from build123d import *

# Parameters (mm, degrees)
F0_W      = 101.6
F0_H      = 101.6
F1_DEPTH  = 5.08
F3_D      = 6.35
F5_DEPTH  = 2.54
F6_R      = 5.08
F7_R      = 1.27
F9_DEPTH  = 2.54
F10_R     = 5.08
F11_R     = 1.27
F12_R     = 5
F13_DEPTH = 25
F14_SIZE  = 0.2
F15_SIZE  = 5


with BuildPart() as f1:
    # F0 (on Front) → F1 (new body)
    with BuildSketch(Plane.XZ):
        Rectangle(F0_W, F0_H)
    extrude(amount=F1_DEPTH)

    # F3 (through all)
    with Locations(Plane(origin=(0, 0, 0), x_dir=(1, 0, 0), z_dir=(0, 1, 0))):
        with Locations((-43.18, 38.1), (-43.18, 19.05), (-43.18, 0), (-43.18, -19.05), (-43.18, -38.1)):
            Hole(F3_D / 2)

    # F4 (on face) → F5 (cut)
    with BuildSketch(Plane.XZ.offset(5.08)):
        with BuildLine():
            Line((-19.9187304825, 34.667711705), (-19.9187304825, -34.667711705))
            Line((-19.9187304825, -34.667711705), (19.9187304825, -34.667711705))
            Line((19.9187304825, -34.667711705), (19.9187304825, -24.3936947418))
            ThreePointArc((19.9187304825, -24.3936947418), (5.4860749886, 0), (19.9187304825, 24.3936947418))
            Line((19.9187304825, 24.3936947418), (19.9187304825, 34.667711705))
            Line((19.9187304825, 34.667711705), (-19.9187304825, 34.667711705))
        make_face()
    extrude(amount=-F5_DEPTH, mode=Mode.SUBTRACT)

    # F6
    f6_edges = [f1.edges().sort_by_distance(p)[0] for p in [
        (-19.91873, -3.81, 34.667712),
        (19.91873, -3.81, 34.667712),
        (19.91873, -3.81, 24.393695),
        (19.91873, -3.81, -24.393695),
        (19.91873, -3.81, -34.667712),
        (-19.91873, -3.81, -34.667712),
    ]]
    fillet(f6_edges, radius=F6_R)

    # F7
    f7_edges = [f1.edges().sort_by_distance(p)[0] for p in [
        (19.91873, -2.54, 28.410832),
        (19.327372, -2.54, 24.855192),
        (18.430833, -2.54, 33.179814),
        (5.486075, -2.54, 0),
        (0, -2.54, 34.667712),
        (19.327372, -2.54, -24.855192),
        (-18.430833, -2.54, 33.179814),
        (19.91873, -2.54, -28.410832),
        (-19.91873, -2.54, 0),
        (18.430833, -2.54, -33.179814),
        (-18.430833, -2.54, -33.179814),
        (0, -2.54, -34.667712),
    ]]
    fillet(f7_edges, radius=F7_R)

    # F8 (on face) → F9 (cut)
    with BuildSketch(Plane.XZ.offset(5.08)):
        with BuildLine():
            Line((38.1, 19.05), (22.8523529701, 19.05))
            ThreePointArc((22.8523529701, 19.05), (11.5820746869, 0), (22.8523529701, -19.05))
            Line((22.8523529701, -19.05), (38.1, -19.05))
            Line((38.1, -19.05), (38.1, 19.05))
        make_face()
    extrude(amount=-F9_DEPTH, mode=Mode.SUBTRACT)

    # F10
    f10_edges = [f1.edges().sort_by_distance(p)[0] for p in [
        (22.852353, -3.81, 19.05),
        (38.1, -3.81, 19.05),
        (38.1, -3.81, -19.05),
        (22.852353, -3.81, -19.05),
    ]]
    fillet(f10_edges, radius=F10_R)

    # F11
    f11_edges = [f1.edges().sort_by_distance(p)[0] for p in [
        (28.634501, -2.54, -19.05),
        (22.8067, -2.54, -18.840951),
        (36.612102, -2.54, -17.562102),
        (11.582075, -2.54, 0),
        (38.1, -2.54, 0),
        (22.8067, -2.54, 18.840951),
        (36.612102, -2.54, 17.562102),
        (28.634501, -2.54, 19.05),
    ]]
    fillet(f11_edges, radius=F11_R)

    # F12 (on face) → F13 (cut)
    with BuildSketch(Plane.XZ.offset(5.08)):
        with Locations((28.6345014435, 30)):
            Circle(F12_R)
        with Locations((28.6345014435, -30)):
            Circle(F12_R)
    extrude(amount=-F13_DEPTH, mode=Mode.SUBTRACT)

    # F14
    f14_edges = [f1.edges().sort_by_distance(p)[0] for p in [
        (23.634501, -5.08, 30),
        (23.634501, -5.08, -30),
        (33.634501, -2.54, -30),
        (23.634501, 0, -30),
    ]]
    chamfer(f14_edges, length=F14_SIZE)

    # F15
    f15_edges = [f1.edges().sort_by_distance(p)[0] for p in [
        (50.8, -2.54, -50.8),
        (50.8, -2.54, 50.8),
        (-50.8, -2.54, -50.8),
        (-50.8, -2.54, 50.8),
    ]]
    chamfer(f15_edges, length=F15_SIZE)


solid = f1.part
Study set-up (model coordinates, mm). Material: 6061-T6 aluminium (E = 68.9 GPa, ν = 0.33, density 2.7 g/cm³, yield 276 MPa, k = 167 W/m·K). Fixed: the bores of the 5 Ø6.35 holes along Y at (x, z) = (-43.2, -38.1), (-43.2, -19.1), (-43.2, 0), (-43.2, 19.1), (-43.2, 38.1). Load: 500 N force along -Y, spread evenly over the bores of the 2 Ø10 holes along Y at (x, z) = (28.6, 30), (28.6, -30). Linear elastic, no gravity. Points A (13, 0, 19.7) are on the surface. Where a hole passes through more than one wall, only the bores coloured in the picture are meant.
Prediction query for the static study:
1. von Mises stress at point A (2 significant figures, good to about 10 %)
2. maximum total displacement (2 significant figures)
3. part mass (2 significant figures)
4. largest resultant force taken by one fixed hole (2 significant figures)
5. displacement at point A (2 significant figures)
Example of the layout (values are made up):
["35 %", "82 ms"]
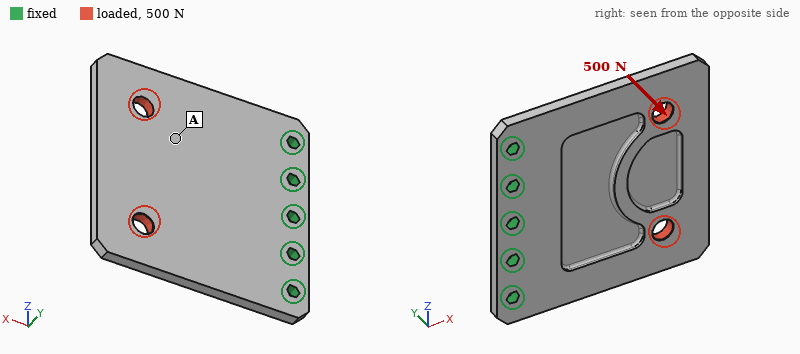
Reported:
["19 MPa", "1.6 mm", "120 g", "660 N", "0.70 mm"]
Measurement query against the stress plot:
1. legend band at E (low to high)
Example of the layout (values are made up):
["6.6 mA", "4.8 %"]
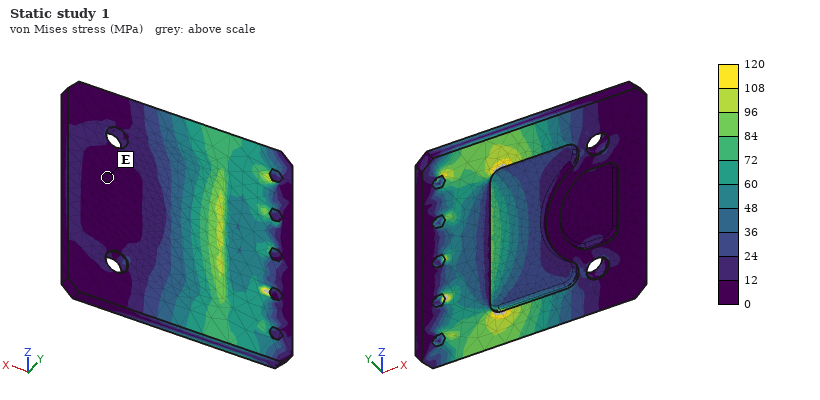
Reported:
["0 to 12 MPa"]
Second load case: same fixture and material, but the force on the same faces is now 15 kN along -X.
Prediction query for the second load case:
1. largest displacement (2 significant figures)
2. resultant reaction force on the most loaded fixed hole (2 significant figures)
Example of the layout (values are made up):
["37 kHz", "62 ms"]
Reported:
["0.66 mm", "4.5 kN"]
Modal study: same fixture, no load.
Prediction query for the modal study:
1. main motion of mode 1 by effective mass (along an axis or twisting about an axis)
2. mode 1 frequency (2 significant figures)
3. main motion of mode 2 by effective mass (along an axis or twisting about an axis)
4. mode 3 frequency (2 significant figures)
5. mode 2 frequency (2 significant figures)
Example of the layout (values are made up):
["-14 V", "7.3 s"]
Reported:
["along Y", "440 Hz", "twisting about X", "2500 Hz", "930 Hz"]
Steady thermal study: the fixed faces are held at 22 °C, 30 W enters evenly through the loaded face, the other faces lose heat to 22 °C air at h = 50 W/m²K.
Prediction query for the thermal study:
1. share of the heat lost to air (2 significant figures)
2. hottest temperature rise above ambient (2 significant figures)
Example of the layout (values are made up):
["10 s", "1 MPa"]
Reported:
["42 %", "24 K"]
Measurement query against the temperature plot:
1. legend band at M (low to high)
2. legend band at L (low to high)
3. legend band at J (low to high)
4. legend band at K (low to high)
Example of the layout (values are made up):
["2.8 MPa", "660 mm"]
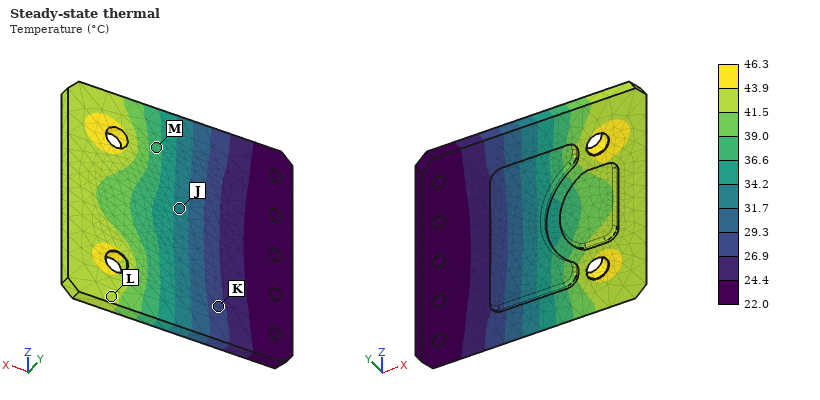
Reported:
["36.6 to 39.0 °C", "41.5 to 43.9 °C", "31.7 to 34.2 °C", "26.9 to 29.3 °C"]
